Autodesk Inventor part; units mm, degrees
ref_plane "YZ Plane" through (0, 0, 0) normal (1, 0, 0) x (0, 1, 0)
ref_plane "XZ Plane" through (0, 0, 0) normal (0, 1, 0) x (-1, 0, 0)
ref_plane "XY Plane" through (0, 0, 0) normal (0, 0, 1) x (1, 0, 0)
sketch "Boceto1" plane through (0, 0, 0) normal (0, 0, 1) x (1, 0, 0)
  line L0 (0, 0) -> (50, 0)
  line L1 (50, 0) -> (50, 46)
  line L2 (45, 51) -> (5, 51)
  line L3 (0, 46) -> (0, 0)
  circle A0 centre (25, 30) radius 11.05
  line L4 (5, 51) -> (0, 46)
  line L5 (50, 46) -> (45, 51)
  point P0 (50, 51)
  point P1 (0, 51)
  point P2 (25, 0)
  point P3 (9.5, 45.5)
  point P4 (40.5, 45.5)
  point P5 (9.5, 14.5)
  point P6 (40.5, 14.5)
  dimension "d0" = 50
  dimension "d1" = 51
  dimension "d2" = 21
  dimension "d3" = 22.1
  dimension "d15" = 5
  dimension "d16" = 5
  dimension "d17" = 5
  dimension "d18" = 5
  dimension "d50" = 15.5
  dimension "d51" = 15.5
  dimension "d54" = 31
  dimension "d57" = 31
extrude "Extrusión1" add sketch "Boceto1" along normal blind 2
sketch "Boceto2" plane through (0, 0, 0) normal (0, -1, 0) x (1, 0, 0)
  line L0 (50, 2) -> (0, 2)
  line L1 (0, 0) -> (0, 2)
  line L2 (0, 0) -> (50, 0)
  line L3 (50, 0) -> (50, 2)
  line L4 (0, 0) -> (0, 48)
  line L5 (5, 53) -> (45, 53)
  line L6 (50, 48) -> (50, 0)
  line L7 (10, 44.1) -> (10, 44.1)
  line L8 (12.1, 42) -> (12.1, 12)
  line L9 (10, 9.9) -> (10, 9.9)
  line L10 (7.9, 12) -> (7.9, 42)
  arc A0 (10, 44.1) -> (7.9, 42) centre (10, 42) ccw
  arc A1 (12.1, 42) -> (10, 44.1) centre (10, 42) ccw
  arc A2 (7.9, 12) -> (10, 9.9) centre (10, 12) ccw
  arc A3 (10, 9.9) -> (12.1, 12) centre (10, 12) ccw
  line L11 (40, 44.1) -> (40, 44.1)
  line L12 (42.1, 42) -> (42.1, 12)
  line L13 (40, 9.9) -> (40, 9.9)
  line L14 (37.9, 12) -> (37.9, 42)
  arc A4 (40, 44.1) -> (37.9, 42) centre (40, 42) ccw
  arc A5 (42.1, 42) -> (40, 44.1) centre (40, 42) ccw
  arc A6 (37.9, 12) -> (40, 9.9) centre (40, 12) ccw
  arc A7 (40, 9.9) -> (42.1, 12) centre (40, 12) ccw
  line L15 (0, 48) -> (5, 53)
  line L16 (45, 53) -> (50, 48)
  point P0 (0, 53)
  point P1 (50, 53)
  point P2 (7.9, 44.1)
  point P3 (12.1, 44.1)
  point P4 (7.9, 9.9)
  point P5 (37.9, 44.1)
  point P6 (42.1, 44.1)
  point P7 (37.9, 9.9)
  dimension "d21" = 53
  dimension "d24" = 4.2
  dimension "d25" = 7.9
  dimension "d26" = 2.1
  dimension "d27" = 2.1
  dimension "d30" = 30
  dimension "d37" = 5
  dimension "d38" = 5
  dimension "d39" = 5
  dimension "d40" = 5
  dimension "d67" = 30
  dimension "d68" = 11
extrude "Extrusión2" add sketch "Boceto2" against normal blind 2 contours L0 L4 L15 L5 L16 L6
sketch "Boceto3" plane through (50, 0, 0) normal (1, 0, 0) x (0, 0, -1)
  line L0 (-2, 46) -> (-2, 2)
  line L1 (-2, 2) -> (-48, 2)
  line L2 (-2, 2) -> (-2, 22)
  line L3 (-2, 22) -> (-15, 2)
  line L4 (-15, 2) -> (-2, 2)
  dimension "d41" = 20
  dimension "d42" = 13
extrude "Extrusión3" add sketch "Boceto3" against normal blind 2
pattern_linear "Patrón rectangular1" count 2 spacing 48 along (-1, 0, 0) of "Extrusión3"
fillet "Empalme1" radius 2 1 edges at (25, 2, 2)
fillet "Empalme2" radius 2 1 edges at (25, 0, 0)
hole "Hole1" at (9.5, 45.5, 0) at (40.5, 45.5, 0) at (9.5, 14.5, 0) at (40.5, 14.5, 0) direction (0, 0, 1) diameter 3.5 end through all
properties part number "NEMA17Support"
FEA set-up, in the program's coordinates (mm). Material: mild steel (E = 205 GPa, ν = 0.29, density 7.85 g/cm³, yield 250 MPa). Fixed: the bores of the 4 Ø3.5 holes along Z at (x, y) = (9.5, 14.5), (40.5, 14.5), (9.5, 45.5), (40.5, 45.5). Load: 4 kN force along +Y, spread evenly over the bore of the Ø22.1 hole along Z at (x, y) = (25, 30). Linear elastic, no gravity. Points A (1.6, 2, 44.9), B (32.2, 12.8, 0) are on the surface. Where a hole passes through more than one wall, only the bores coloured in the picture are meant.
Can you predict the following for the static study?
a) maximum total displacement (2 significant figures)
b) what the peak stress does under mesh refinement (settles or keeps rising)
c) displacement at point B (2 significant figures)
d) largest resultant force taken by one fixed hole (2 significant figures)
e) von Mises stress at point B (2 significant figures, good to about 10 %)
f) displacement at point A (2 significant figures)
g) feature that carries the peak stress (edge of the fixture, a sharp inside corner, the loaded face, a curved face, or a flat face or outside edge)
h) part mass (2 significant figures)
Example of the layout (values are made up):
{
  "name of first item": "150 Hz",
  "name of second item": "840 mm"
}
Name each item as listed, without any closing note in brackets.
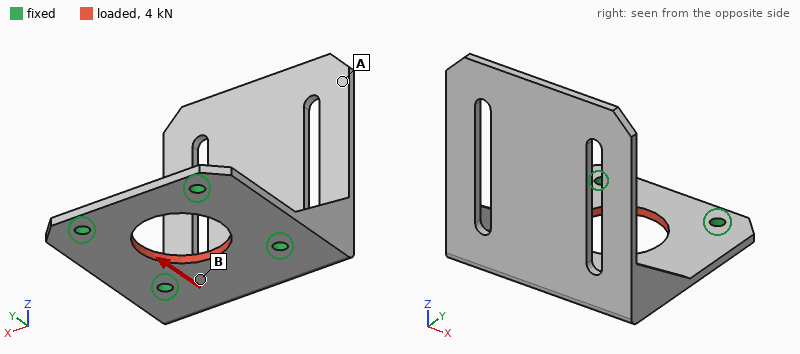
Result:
{
  "maximum total displacement": "6.0 µm",
  "what the peak stress does under mesh refinement": "keeps rising",
  "displacement at point B": "2.0 µm",
  "largest resultant force taken by one fixed hole": "1.0 kN",
  "von Mises stress at point B": "22 MPa",
  "displacement at point A": "2.6 µm",
  "feature that carries the peak stress": "edge of the fixture",
  "part mass": "72 g"
}
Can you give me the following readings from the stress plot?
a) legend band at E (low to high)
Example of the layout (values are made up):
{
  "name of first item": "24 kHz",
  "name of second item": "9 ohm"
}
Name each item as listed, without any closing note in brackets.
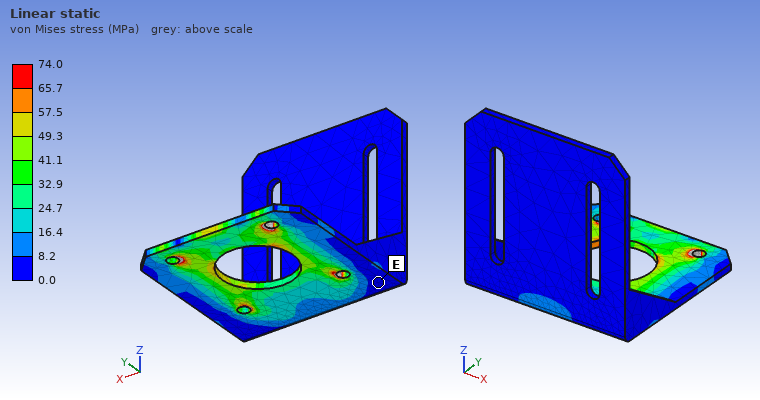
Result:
{
  "legend band at E": "0.0 to 8.2 MPa"
}
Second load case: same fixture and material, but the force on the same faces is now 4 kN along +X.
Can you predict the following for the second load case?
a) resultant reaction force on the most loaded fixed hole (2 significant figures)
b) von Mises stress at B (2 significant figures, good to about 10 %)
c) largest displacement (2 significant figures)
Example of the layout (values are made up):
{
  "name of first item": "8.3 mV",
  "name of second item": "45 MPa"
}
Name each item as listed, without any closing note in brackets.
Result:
{
  "resultant reaction force on the most loaded fixed hole": "1.0 kN",
  "von Mises stress at B": "23 MPa",
  "largest displacement": "4.6 µm"
}
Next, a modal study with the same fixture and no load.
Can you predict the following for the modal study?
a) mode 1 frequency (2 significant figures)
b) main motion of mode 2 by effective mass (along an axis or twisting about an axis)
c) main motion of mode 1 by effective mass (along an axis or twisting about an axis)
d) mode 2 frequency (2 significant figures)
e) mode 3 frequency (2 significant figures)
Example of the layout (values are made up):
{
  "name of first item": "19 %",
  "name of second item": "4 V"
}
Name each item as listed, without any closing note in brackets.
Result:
{
  "mode 1 frequency": "640 Hz",
  "main motion of mode 2 by effective mass": "along X",
  "main motion of mode 1 by effective mass": "along Y",
  "mode 2 frequency": "1500 Hz",
  "mode 3 frequency": "2300 Hz"
}
